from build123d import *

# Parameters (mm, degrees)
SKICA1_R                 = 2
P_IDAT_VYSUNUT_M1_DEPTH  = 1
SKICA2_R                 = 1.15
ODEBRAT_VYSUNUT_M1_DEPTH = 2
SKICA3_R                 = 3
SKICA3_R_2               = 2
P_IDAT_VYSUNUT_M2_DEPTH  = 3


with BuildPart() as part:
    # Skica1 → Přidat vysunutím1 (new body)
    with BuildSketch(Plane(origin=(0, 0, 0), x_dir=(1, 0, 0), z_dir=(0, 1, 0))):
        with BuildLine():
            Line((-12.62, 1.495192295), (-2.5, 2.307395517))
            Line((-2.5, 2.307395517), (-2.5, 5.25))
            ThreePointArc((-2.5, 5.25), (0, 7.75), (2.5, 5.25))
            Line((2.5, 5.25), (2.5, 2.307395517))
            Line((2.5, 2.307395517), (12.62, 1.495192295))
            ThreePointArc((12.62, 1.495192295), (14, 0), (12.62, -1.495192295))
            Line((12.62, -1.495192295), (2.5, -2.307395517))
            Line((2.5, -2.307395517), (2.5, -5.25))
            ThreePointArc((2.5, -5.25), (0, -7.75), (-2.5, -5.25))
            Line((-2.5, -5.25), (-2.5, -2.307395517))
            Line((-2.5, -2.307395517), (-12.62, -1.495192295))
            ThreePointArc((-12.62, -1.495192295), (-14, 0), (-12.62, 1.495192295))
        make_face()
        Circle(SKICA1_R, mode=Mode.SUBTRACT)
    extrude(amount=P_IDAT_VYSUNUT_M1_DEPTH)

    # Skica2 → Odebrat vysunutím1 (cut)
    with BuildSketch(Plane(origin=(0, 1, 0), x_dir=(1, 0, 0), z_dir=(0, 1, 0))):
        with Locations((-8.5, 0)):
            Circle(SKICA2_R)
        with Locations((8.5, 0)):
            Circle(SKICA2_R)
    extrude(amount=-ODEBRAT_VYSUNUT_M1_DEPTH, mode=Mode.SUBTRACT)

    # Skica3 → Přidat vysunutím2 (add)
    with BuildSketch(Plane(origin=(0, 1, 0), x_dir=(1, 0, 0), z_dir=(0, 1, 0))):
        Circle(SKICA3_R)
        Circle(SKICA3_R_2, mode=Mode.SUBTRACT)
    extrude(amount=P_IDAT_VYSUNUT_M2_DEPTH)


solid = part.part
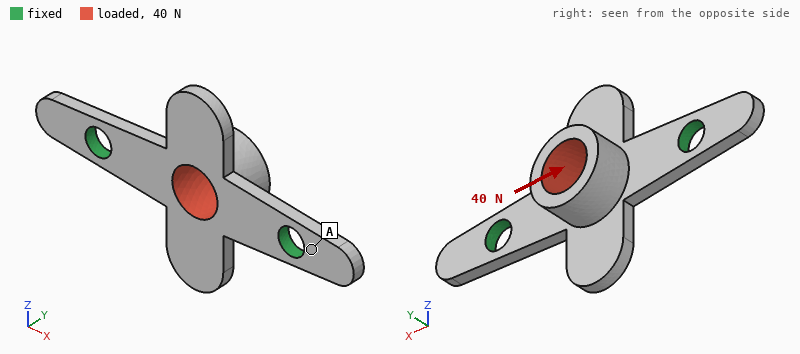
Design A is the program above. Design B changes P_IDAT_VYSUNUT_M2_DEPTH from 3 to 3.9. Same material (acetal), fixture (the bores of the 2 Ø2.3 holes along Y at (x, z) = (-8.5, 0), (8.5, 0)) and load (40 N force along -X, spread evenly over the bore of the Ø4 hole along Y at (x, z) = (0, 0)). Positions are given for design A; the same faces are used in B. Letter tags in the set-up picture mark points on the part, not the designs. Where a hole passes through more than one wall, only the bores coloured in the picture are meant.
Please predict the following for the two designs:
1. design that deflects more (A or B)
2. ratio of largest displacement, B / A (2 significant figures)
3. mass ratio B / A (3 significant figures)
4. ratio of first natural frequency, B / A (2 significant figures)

B
1.5
1.08
0.93
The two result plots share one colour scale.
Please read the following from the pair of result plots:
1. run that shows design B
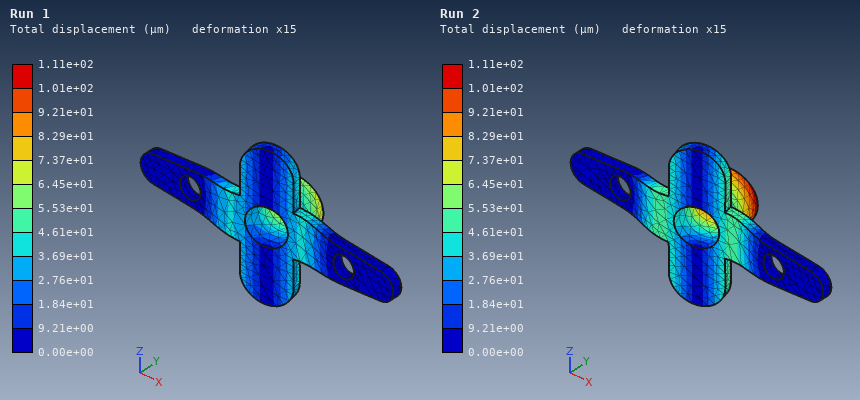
Run 2
